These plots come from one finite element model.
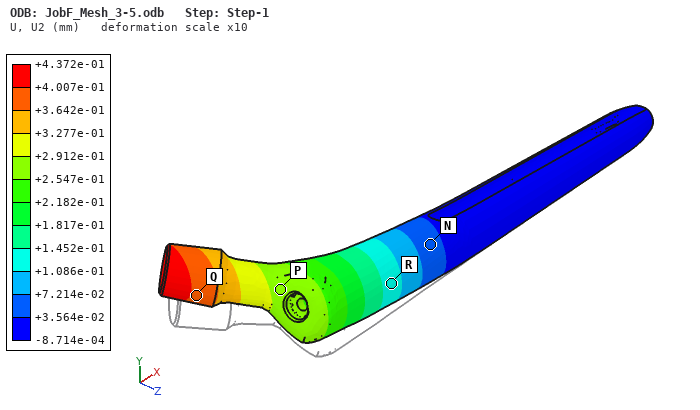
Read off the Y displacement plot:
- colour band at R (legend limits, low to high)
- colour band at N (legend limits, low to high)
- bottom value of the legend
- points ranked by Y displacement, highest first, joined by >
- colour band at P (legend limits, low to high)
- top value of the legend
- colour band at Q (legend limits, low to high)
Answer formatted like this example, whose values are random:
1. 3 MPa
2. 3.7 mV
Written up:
1. +1.086e-01 to +1.452e-01 mm
2. +3.564e-02 to +7.214e-02 mm
3. -8.714e-04 mm
4. Q > P > R > N
5. +2.547e-01 to +2.912e-01 mm
6. +4.372e-01 mm
7. +3.642e-01 to +4.007e-01 mm
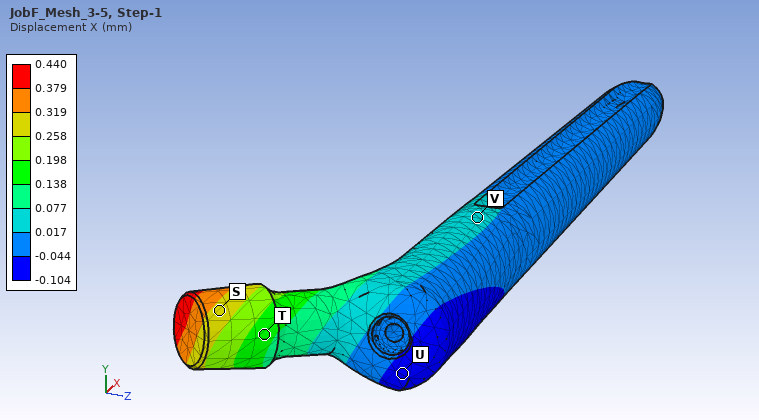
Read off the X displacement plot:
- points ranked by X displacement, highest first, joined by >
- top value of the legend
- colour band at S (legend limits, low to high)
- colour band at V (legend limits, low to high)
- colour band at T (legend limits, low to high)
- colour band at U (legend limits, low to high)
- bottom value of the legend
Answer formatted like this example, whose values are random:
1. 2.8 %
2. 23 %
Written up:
1. S > T > V > U
2. 0.440 mm
3. 0.258 to 0.319 mm
4. 0.017 to 0.077 mm
5. 0.138 to 0.198 mm
6. -0.104 to -0.044 mm
7. -0.104 mm
